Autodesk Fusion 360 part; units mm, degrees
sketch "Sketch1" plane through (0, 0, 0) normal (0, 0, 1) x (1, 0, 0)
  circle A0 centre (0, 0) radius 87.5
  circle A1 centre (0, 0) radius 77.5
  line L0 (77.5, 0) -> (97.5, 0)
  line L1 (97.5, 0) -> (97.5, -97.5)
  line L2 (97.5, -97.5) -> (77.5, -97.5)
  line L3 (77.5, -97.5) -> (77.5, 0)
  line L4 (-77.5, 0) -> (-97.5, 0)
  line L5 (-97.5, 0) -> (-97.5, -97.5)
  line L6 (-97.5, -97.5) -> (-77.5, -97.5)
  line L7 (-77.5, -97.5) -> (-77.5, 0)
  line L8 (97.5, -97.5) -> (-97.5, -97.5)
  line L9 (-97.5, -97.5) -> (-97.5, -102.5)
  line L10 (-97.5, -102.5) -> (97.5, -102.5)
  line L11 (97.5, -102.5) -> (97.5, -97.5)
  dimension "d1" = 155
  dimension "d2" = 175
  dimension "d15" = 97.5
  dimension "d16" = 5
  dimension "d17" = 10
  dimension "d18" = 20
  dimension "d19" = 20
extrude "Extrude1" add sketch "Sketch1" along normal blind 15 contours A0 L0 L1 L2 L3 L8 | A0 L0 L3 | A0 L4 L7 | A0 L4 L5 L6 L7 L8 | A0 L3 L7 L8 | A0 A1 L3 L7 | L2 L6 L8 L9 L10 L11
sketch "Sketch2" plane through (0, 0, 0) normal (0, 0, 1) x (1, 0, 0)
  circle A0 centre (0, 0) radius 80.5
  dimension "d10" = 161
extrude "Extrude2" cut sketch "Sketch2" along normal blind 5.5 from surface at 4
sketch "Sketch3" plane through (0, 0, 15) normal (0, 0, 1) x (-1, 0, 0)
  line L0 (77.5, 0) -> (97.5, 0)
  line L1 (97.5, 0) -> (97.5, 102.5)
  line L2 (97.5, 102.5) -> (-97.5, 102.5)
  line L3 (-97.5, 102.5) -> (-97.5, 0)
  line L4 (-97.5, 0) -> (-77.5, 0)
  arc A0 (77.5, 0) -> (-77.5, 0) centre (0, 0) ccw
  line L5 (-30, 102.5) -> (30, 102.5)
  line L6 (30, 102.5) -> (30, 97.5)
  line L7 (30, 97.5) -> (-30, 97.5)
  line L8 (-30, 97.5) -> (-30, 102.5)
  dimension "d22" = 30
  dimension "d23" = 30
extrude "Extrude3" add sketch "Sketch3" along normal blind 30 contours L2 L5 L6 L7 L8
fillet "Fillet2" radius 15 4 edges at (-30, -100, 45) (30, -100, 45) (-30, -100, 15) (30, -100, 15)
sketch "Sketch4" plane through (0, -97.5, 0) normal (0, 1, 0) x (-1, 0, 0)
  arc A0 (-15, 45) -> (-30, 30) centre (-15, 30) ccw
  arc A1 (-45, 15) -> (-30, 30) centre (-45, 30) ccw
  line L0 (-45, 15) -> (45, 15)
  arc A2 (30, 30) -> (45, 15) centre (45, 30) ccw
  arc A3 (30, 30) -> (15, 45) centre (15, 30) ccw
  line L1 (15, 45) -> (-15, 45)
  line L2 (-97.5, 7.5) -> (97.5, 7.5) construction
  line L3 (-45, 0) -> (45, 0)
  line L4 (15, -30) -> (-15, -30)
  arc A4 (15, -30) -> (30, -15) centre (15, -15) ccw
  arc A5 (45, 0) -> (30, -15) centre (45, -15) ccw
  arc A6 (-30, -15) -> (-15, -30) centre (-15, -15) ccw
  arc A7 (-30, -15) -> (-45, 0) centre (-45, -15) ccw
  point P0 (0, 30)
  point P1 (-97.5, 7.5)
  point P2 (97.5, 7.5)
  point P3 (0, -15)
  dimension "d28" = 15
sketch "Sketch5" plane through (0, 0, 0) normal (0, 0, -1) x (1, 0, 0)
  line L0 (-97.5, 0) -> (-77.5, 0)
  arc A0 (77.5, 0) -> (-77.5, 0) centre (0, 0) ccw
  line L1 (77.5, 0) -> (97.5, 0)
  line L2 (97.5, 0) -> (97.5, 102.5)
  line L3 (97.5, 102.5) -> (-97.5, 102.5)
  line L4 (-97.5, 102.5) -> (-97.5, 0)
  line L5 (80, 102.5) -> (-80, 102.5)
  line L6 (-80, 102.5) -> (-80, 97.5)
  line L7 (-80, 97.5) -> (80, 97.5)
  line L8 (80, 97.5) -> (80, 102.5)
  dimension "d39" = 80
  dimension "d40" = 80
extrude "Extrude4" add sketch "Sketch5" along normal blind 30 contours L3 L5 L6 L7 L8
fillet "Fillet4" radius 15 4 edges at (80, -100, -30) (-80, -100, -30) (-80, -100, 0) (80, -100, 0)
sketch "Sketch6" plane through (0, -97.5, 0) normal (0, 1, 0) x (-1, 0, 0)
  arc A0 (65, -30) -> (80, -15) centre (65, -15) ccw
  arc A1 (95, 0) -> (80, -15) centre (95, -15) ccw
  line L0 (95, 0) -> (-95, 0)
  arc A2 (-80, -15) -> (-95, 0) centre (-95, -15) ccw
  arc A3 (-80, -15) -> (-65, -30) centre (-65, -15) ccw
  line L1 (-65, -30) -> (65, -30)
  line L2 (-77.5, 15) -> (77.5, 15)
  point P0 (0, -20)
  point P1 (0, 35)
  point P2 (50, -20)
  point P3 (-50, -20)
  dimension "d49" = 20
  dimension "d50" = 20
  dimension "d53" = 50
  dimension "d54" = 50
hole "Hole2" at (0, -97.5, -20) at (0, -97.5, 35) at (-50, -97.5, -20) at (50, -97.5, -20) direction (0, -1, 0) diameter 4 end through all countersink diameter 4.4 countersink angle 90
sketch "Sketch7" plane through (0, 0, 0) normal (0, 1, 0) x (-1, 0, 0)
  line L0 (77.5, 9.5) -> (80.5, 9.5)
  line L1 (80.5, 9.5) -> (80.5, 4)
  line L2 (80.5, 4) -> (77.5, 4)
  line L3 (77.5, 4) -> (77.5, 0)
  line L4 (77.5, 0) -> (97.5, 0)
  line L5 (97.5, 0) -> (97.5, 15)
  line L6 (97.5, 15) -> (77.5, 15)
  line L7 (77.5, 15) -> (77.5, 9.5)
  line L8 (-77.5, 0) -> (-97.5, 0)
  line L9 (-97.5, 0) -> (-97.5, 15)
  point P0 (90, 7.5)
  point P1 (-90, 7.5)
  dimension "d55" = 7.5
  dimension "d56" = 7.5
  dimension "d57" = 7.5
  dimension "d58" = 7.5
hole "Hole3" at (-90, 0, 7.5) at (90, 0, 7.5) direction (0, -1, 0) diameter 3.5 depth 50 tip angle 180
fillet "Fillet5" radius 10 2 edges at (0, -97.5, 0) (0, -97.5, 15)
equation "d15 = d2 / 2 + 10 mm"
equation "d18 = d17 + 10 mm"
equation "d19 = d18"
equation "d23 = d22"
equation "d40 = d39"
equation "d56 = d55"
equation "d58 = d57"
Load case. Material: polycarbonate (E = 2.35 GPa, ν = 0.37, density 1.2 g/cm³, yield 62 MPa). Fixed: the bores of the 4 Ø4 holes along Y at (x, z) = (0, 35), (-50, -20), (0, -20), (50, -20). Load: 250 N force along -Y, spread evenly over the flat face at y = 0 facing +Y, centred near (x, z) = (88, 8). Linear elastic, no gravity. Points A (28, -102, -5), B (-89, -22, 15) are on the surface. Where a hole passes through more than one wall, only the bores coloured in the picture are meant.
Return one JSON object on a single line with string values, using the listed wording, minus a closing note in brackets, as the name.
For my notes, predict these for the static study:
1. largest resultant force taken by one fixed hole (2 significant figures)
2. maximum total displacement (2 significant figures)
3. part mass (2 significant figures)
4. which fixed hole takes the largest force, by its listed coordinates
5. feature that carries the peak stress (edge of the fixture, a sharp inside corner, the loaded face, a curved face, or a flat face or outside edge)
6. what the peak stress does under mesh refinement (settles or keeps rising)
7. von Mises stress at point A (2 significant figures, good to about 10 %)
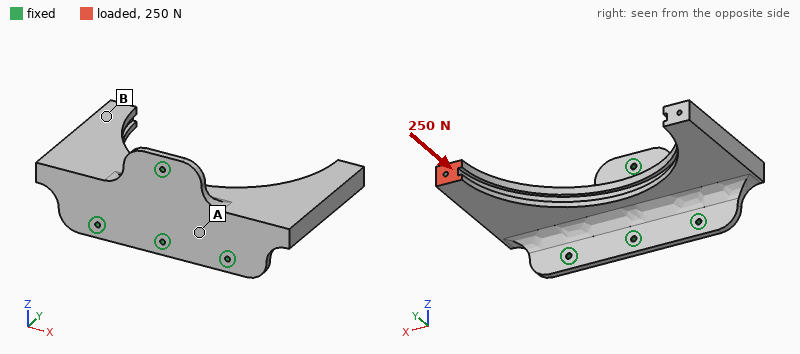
{"largest resultant force taken by one fixed hole": "290 N", "maximum total displacement": "1.9 mm", "part mass": "230 g", "which fixed hole takes the largest force, by its listed coordinates": "(50, -20)", "feature that carries the peak stress": "edge of the fixture", "what the peak stress does under mesh refinement": "keeps rising", "von Mises stress at point A": "3.9 MPa"}
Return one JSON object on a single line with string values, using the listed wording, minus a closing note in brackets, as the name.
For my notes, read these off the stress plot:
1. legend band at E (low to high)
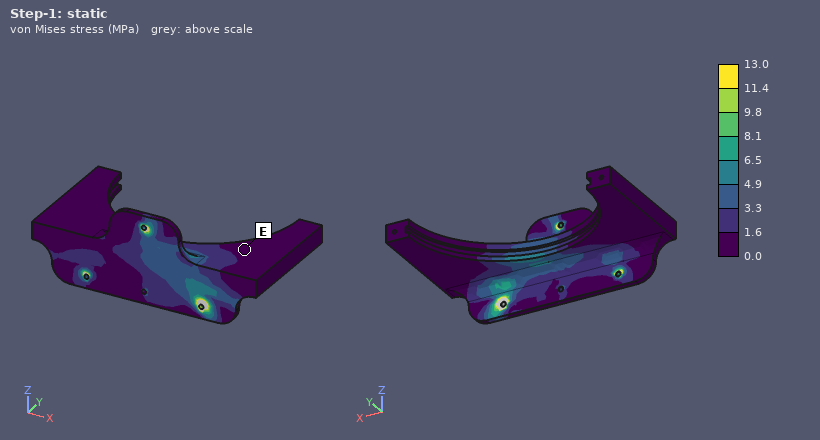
{"legend band at E": "0.0 to 1.6 MPa"}
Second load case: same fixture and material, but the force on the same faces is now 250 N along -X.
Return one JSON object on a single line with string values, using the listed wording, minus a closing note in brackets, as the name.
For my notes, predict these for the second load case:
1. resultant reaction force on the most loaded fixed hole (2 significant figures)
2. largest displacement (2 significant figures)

{"resultant reaction force on the most loaded fixed hole": "290 N", "largest displacement": "2.6 mm"}
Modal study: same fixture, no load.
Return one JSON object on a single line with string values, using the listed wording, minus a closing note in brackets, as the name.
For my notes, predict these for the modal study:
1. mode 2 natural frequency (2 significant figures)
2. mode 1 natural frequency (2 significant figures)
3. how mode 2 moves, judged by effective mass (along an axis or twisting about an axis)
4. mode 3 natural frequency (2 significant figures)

{"mode 2 natural frequency": "240 Hz", "mode 1 natural frequency": "210 Hz", "how mode 2 moves, judged by effective mass": "along Z", "mode 3 natural frequency": "390 Hz"}
